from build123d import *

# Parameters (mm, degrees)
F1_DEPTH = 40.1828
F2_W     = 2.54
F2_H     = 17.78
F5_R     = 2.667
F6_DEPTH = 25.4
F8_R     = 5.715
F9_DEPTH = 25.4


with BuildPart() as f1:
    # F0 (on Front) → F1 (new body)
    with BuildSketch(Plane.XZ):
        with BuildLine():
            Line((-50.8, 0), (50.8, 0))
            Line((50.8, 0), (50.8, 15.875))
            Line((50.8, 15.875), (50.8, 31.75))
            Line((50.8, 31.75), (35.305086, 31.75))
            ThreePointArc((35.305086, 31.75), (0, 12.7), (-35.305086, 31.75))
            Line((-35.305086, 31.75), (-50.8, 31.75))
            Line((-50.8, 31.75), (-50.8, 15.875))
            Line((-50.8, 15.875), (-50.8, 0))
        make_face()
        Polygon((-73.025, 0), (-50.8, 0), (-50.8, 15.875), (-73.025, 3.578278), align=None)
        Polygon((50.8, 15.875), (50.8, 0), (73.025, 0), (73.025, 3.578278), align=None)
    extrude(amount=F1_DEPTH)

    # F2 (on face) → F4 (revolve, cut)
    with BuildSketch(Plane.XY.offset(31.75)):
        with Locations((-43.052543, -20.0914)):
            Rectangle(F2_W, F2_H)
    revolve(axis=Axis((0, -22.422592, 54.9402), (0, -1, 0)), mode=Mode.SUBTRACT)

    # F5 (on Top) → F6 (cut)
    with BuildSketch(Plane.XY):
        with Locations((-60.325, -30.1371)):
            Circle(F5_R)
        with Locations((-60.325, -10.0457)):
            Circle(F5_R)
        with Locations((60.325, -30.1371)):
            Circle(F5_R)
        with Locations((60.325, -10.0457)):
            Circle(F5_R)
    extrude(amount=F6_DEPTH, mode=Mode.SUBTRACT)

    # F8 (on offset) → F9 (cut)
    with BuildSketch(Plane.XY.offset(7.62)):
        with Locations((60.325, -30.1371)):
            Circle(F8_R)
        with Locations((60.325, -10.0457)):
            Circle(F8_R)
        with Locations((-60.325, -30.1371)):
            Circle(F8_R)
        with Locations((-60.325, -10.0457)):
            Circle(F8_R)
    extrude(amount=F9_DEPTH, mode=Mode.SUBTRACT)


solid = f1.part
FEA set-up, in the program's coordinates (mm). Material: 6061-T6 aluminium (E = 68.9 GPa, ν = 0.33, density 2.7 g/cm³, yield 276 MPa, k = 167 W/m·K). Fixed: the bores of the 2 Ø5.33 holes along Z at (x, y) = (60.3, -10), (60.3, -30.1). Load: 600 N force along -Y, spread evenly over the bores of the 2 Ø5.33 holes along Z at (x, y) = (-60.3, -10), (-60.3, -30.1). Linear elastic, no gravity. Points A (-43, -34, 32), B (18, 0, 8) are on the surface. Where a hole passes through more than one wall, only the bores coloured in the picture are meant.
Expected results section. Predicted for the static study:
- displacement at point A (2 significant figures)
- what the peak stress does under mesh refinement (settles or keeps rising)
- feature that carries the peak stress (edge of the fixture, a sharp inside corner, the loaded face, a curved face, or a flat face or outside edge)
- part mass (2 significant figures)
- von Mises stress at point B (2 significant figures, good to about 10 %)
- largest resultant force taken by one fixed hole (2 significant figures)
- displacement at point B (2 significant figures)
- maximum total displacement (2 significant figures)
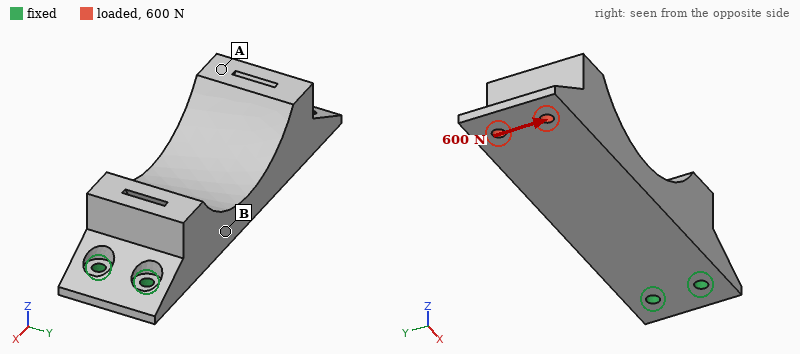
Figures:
0.072 mm
keeps rising
edge of the fixture
280 g
12 MPa
3.1 kN
0.027 mm
0.12 mm
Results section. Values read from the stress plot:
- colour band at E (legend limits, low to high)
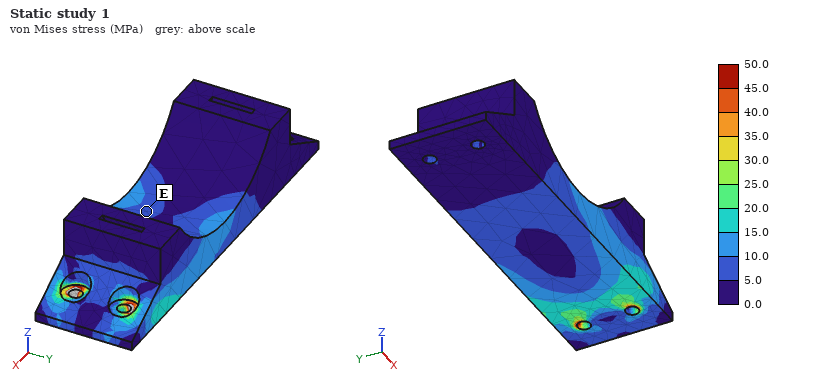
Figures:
5.0 to 10.0 MPa
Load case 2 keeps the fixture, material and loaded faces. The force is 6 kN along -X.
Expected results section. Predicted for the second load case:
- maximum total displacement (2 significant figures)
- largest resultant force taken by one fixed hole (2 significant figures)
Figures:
0.20 mm
3.0 kN
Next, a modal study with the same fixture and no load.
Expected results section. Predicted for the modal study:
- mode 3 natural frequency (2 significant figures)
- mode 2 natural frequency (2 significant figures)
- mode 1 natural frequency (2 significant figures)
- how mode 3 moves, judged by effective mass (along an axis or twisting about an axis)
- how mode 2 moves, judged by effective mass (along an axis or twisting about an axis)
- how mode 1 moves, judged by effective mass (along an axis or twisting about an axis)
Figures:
3300 Hz
1400 Hz
500 Hz
twisting about X
along Y
along Z
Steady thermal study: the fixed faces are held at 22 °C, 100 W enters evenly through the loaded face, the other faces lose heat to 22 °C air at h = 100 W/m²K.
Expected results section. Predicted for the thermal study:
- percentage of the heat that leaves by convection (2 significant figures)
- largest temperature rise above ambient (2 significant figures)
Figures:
66 %
73 K
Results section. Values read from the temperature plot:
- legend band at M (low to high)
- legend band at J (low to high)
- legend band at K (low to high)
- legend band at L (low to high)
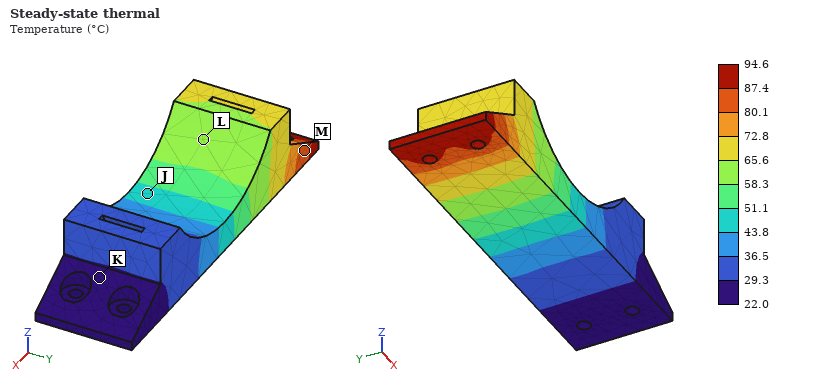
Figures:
80.1 to 87.4 °C
43.8 to 51.1 °C
22.0 to 29.3 °C
58.3 to 65.6 °C
